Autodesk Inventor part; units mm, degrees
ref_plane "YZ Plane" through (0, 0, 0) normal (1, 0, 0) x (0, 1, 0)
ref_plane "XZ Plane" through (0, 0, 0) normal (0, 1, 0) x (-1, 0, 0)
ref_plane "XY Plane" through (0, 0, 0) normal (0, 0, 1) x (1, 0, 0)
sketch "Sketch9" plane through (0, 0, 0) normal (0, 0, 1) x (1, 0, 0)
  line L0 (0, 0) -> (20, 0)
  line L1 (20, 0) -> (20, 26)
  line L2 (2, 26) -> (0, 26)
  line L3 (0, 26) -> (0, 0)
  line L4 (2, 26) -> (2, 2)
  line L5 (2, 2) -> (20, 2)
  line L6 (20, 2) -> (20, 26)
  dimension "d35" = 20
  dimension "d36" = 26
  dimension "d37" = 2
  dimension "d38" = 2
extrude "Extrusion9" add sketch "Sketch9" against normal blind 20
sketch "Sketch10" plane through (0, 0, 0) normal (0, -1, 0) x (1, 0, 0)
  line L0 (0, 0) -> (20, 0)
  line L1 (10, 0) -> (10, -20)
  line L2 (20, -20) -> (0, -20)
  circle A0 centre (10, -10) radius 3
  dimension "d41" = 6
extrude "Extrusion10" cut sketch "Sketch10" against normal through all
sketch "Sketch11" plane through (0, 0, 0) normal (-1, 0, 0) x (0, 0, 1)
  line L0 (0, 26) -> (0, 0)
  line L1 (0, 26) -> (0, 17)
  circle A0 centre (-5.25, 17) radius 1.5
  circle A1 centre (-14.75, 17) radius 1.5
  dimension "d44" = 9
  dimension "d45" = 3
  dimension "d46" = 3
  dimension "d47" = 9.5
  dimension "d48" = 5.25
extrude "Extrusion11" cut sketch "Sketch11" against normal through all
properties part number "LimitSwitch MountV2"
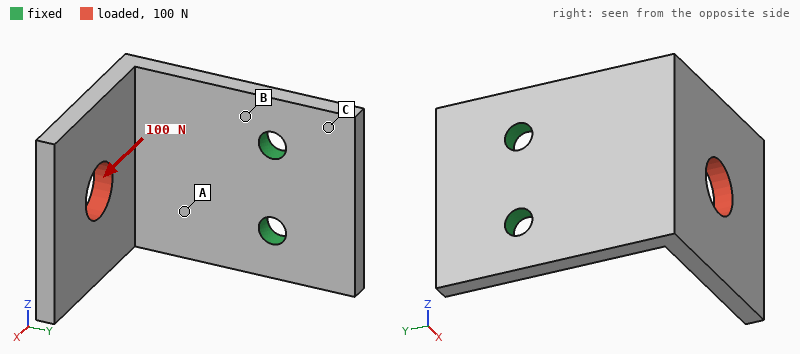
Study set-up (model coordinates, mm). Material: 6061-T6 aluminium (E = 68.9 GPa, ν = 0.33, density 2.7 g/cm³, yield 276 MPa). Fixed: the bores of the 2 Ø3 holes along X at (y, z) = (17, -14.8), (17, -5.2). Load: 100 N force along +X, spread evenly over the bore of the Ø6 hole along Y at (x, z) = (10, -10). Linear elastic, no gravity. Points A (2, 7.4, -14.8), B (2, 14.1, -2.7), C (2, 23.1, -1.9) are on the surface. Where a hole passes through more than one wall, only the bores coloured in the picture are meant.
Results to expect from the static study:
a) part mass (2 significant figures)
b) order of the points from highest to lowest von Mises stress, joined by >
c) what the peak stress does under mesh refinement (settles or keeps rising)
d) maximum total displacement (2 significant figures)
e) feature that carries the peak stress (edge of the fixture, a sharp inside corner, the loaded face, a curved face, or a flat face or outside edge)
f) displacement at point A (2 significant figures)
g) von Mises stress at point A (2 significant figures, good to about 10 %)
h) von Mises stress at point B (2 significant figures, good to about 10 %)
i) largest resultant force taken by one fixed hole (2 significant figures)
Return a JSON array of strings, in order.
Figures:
["4.5 g", "B > A > C", "keeps rising", "0.27 mm", "edge of the fixture", "0.053 mm", "43 MPa", "83 MPa", "50 N"]
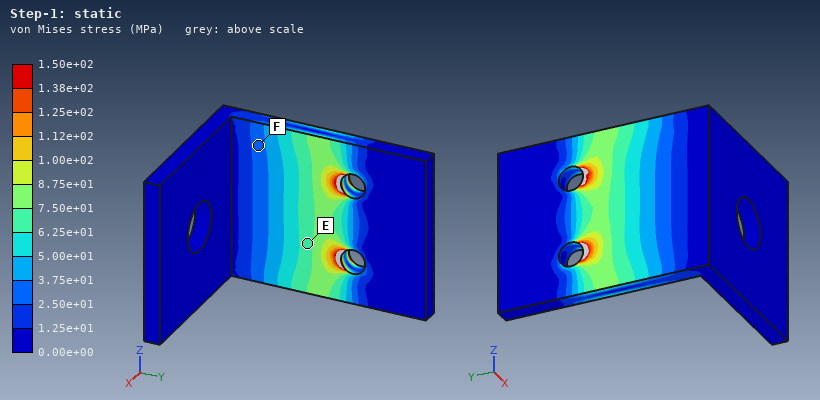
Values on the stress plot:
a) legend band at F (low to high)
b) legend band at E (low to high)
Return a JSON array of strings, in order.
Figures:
["2.50e+01 to 3.75e+01 MPa", "6.25e+01 to 7.50e+01 MPa"]
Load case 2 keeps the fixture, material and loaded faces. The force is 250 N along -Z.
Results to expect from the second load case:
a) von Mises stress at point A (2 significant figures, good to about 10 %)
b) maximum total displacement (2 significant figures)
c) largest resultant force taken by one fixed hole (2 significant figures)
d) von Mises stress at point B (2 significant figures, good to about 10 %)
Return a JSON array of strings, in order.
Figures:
["120 MPa", "0.34 mm", "400 N", "96 MPa"]
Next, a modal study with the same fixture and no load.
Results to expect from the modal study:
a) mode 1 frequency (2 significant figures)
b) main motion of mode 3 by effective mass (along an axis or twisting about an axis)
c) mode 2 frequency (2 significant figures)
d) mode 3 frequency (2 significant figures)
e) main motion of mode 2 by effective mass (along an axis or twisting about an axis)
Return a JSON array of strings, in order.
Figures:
["1900 Hz", "along X", "3400 Hz", "5300 Hz", "along Z"]
